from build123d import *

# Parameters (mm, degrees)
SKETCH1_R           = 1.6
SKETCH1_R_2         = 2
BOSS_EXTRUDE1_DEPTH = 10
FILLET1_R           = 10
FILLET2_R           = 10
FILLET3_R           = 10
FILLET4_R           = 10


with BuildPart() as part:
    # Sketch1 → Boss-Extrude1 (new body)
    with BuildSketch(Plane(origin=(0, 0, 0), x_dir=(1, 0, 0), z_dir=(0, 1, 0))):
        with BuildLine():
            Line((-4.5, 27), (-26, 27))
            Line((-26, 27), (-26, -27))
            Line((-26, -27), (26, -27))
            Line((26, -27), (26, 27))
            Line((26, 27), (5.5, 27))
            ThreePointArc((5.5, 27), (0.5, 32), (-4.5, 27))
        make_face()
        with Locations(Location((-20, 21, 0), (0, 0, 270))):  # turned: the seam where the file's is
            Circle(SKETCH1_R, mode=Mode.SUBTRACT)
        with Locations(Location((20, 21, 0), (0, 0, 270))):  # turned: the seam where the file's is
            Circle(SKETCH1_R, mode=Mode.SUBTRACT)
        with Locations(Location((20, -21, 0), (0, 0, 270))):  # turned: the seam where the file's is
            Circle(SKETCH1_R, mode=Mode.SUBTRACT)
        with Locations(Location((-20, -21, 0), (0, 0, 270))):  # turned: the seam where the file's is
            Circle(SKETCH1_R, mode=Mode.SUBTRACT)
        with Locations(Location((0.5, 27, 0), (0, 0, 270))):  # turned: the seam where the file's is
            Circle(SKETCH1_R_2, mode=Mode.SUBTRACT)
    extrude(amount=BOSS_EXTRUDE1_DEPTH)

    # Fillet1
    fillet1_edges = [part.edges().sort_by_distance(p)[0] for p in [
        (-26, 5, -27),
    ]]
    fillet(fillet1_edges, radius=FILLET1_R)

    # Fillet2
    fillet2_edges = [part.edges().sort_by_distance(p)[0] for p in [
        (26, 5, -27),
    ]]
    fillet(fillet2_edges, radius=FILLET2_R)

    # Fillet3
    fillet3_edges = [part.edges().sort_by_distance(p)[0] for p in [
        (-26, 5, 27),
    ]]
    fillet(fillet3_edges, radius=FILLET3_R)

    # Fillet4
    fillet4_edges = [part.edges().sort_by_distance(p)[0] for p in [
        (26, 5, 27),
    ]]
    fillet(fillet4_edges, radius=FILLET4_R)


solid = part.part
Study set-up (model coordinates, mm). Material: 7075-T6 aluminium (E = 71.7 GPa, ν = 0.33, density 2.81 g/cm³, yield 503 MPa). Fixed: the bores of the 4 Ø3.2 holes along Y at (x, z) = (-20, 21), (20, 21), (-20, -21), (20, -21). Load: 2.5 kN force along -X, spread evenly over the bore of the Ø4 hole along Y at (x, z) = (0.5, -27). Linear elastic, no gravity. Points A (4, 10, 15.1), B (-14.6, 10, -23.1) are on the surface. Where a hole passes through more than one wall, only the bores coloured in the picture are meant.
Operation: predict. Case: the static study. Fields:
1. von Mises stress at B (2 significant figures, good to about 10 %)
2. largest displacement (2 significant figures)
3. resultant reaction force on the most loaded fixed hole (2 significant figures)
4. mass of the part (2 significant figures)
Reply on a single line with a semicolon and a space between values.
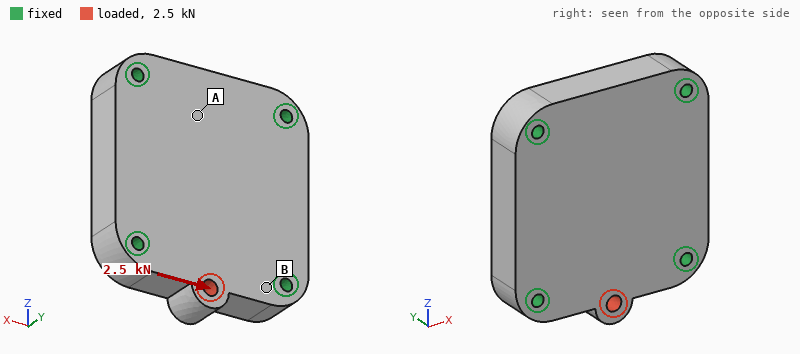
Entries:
15 MPa; 8.1 µm; 1.3 kN; 76 g
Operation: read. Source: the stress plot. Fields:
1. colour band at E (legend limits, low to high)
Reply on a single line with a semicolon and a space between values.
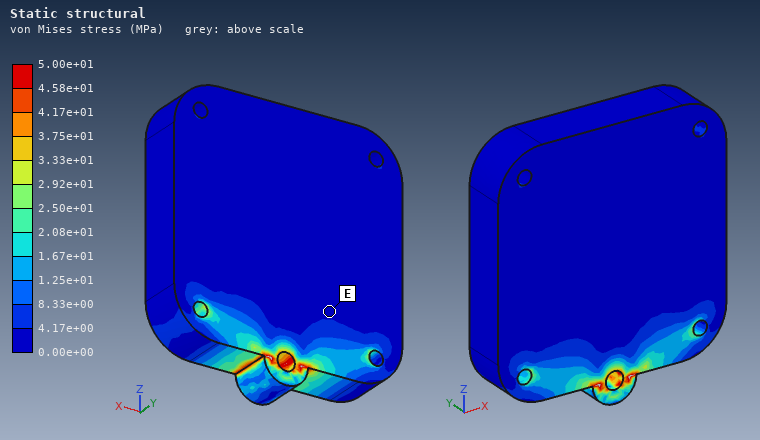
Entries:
0.00e+00 to 4.17e+00 MPa
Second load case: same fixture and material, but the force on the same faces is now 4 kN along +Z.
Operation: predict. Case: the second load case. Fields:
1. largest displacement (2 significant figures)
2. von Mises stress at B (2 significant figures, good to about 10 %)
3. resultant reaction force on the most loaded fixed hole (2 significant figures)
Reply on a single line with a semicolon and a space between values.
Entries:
11 µm; 6.9 MPa; 1.2 kN
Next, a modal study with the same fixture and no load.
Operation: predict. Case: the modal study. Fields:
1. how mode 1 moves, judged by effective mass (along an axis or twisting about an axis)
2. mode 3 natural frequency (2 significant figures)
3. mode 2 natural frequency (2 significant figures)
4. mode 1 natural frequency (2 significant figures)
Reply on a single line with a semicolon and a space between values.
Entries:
along Y; 23 kHz; 22 kHz; 15 kHz
